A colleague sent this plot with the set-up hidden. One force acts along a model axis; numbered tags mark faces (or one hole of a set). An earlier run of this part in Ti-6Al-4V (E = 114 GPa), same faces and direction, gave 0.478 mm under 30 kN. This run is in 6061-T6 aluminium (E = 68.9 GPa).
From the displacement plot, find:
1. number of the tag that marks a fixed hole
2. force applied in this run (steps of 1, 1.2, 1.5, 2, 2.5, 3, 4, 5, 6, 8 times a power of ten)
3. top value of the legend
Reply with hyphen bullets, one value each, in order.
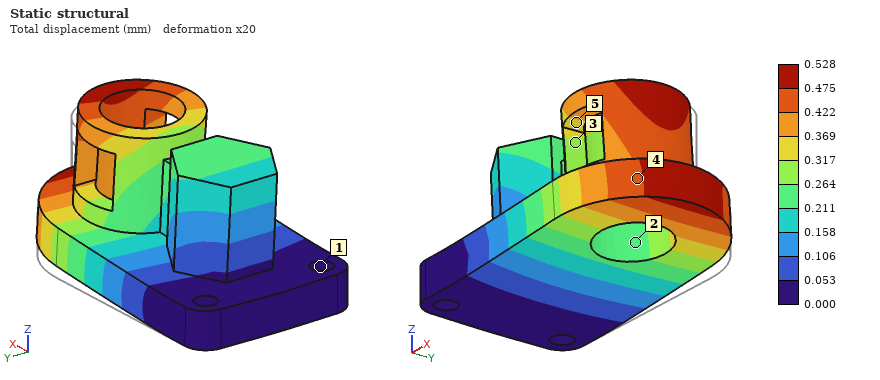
- 1
- 20 kN
- 0.528 mm
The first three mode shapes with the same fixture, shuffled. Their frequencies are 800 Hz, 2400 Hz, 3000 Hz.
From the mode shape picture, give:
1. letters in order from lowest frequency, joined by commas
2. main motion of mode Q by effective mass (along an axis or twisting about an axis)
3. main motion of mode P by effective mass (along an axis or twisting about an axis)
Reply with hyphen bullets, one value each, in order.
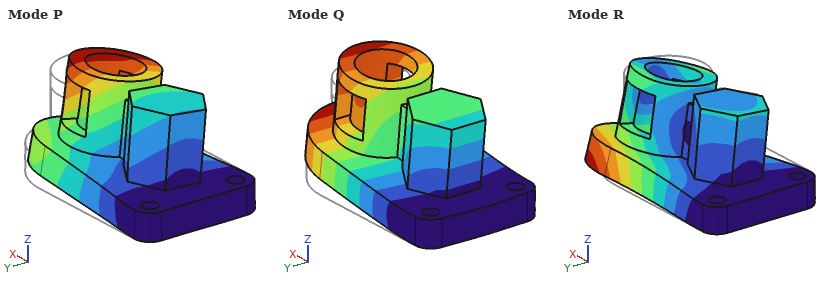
- Q, P, R
- along Z
- along Y
